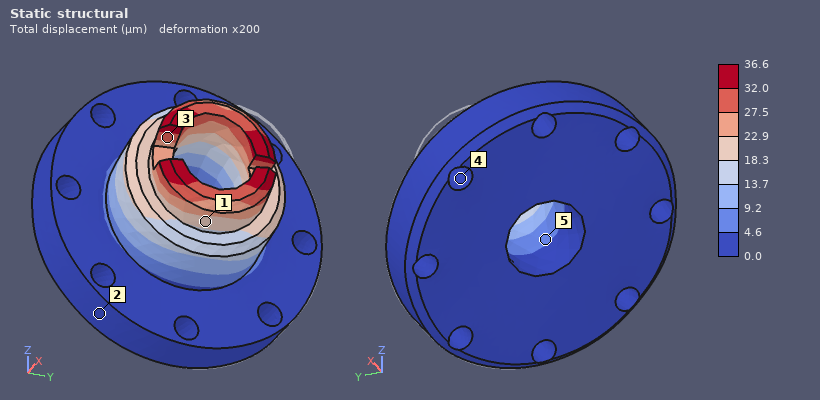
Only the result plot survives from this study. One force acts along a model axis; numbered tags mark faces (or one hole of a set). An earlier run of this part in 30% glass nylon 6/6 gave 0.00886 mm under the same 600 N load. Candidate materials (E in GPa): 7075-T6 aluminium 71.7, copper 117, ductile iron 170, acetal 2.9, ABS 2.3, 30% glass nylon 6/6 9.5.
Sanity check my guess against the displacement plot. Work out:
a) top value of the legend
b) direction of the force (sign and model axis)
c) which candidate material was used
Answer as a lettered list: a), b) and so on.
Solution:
a) 36.6 µm
b) -Y
c) ABS
